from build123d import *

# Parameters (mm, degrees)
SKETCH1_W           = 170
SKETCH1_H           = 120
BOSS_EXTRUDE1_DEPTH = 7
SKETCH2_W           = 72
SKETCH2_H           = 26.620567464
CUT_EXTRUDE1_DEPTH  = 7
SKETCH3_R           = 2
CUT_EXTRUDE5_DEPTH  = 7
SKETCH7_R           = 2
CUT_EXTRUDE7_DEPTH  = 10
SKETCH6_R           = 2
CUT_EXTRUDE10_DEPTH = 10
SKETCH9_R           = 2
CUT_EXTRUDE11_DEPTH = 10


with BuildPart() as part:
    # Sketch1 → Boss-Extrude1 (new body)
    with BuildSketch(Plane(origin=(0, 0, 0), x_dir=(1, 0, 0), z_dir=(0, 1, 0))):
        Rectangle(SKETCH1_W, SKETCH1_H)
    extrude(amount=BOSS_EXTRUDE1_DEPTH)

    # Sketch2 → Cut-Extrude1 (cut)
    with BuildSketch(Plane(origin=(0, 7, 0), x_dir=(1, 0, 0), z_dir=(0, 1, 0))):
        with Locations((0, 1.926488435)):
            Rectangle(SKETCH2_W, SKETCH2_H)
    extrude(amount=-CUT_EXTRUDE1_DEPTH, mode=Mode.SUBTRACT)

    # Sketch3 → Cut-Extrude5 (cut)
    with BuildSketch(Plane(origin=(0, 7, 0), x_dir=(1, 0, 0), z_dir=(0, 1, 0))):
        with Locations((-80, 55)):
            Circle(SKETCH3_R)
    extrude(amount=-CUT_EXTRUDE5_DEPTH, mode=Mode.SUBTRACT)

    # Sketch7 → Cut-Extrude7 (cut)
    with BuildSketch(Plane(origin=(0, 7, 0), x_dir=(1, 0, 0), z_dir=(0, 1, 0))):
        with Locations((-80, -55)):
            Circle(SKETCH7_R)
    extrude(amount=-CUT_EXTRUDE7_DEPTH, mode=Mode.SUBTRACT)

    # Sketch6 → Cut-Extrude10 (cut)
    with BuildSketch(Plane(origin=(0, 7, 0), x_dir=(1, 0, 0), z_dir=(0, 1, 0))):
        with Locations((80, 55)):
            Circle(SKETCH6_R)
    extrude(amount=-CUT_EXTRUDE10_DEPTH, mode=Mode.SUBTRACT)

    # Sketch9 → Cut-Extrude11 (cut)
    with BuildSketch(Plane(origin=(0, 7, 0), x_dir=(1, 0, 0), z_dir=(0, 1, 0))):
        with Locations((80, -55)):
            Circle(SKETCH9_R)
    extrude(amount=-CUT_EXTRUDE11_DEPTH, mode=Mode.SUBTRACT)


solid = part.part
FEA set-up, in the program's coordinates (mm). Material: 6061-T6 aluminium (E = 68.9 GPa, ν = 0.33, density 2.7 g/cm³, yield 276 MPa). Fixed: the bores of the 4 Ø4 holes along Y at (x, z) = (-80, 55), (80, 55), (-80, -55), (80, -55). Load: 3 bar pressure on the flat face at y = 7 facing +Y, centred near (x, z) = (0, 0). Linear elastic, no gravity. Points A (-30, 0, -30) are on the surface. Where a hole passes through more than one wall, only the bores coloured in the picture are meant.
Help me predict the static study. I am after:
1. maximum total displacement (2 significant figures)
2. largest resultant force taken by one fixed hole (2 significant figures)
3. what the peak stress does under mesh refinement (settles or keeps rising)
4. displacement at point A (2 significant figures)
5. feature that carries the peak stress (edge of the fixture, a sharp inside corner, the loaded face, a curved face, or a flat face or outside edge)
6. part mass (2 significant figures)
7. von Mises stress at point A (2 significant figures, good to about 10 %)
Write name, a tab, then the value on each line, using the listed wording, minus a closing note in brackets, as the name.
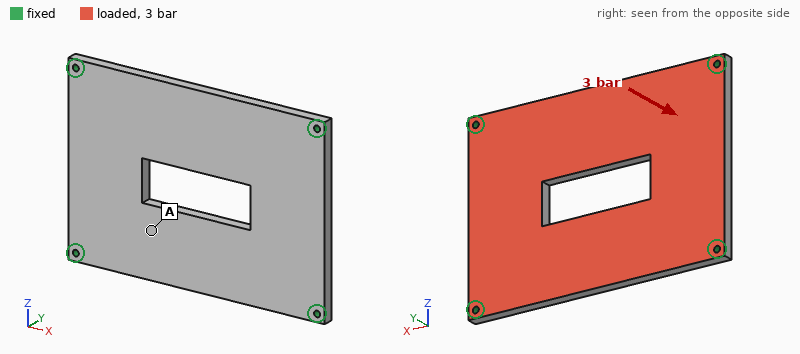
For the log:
maximum total displacement	0.63 mm
largest resultant force taken by one fixed hole	1.4 kN
what the peak stress does under mesh refinement	keeps rising
displacement at point A	0.45 mm
feature that carries the peak stress	edge of the fixture
part mass	350 g
von Mises stress at point A	38 MPa
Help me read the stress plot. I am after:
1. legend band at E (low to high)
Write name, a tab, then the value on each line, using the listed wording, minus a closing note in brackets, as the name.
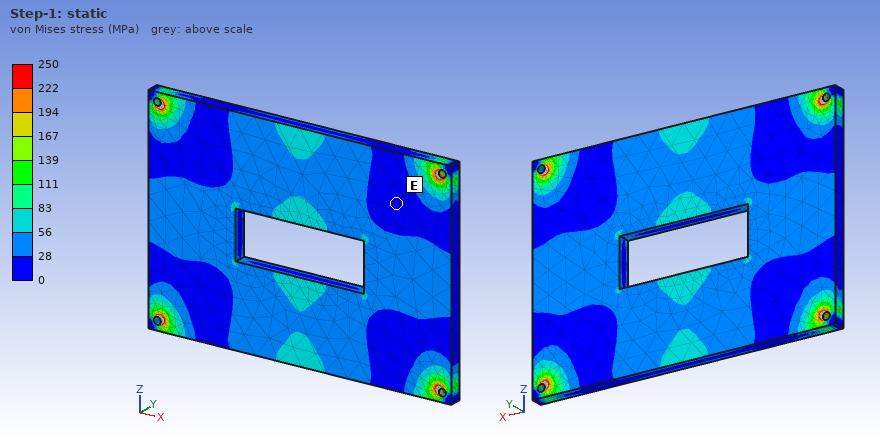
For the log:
legend band at E	0 to 28 MPa
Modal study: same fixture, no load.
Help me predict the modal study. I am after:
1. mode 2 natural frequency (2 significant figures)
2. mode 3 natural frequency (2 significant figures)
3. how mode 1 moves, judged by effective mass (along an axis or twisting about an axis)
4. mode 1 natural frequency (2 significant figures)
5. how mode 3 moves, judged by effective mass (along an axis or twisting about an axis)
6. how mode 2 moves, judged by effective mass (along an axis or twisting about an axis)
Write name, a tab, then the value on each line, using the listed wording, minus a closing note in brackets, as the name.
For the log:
mode 2 natural frequency	1600 Hz
mode 3 natural frequency	2300 Hz
how mode 1 moves, judged by effective mass	along Y
mode 1 natural frequency	1000 Hz
how mode 3 moves, judged by effective mass	twisting about Z
how mode 2 moves, judged by effective mass	twisting about X
